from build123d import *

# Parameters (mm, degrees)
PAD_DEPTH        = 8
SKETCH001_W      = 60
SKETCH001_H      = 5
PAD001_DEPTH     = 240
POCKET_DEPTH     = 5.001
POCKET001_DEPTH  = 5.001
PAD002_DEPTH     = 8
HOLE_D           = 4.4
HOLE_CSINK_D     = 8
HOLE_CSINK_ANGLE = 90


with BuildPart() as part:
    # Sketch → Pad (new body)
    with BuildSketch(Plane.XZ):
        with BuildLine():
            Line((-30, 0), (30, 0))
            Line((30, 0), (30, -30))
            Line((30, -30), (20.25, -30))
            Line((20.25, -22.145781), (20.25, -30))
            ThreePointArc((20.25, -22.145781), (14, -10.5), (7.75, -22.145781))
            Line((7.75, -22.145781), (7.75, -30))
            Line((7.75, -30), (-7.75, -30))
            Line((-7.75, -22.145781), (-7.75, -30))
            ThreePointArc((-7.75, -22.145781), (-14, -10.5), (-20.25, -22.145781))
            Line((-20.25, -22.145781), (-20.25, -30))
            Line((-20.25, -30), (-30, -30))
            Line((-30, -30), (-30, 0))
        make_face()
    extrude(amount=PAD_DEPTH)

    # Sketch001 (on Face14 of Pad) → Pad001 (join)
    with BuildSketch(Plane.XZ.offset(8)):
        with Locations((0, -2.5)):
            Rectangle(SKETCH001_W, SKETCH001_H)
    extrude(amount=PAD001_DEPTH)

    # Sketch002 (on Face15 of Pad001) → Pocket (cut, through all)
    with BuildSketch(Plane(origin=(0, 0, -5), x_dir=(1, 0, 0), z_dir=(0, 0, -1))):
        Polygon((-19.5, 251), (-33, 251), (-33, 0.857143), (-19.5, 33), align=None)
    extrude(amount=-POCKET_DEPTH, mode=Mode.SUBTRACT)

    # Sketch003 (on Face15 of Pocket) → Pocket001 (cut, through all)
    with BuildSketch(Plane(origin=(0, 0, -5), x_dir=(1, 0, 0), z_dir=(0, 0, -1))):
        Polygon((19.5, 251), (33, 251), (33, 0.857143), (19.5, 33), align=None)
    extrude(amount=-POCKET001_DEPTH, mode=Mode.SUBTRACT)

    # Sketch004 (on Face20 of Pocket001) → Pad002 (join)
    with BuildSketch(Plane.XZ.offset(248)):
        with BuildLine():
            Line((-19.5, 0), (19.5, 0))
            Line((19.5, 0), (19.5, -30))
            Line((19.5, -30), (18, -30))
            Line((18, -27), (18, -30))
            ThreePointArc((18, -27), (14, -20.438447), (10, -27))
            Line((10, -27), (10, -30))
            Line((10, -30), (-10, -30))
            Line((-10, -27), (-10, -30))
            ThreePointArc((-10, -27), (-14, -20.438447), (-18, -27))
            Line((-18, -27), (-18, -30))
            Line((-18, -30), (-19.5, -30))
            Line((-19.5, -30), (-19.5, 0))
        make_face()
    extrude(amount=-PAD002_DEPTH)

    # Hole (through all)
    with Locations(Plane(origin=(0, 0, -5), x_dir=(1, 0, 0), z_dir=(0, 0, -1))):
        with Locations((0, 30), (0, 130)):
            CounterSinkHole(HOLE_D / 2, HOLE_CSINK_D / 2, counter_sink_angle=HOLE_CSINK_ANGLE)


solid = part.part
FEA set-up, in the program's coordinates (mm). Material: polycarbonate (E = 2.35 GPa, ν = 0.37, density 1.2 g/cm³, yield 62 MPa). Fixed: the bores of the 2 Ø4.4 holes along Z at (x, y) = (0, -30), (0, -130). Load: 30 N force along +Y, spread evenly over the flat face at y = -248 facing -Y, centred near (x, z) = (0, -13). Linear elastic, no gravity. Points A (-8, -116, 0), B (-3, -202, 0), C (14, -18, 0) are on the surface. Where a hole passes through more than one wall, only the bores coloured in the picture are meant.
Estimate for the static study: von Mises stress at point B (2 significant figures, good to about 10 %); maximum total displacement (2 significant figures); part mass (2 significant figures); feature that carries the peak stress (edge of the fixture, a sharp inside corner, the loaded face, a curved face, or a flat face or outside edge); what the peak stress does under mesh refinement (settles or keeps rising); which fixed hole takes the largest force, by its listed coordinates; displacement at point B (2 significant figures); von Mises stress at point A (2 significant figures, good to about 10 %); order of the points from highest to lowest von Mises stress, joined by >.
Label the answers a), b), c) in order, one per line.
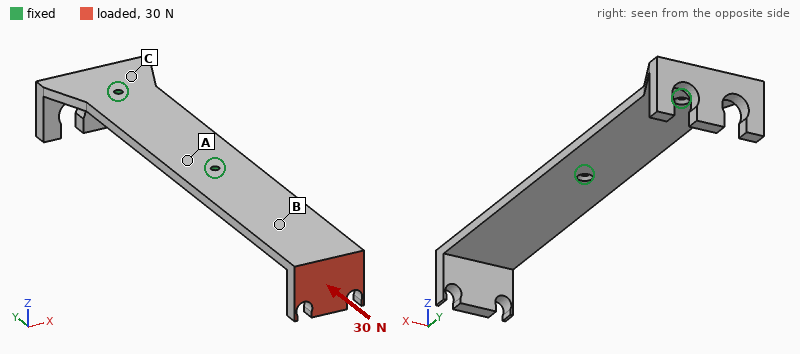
a) 1.8 MPa
b) 2.8 mm
c) 78 g
d) edge of the fixture
e) keeps rising
f) (0, -130)
g) 1.0 mm
h) 0.48 MPa
i) B > A > C
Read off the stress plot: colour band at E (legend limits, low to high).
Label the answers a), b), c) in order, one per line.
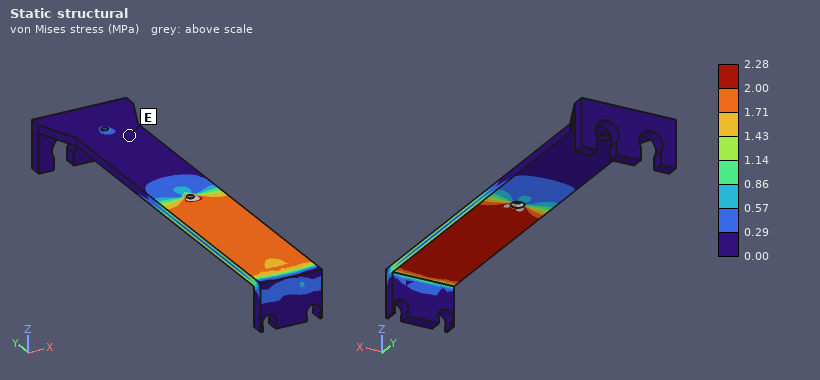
a) 0.00 to 0.29 MPa
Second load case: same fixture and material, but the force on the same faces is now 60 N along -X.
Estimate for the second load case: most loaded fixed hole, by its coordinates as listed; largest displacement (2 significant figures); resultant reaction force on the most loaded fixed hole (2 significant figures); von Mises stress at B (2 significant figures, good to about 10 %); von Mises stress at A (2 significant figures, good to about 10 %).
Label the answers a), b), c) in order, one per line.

a) (0, -130)
b) 3.0 mm
c) 120 N
d) 3.0 MPa
e) 2.2 MPa
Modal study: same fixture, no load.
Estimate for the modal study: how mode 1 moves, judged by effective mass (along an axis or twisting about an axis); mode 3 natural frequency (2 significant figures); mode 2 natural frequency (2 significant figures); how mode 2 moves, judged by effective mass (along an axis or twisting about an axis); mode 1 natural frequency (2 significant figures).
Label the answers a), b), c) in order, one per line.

a) along Z
b) 350 Hz
c) 230 Hz
d) along X
e) 52 Hz
